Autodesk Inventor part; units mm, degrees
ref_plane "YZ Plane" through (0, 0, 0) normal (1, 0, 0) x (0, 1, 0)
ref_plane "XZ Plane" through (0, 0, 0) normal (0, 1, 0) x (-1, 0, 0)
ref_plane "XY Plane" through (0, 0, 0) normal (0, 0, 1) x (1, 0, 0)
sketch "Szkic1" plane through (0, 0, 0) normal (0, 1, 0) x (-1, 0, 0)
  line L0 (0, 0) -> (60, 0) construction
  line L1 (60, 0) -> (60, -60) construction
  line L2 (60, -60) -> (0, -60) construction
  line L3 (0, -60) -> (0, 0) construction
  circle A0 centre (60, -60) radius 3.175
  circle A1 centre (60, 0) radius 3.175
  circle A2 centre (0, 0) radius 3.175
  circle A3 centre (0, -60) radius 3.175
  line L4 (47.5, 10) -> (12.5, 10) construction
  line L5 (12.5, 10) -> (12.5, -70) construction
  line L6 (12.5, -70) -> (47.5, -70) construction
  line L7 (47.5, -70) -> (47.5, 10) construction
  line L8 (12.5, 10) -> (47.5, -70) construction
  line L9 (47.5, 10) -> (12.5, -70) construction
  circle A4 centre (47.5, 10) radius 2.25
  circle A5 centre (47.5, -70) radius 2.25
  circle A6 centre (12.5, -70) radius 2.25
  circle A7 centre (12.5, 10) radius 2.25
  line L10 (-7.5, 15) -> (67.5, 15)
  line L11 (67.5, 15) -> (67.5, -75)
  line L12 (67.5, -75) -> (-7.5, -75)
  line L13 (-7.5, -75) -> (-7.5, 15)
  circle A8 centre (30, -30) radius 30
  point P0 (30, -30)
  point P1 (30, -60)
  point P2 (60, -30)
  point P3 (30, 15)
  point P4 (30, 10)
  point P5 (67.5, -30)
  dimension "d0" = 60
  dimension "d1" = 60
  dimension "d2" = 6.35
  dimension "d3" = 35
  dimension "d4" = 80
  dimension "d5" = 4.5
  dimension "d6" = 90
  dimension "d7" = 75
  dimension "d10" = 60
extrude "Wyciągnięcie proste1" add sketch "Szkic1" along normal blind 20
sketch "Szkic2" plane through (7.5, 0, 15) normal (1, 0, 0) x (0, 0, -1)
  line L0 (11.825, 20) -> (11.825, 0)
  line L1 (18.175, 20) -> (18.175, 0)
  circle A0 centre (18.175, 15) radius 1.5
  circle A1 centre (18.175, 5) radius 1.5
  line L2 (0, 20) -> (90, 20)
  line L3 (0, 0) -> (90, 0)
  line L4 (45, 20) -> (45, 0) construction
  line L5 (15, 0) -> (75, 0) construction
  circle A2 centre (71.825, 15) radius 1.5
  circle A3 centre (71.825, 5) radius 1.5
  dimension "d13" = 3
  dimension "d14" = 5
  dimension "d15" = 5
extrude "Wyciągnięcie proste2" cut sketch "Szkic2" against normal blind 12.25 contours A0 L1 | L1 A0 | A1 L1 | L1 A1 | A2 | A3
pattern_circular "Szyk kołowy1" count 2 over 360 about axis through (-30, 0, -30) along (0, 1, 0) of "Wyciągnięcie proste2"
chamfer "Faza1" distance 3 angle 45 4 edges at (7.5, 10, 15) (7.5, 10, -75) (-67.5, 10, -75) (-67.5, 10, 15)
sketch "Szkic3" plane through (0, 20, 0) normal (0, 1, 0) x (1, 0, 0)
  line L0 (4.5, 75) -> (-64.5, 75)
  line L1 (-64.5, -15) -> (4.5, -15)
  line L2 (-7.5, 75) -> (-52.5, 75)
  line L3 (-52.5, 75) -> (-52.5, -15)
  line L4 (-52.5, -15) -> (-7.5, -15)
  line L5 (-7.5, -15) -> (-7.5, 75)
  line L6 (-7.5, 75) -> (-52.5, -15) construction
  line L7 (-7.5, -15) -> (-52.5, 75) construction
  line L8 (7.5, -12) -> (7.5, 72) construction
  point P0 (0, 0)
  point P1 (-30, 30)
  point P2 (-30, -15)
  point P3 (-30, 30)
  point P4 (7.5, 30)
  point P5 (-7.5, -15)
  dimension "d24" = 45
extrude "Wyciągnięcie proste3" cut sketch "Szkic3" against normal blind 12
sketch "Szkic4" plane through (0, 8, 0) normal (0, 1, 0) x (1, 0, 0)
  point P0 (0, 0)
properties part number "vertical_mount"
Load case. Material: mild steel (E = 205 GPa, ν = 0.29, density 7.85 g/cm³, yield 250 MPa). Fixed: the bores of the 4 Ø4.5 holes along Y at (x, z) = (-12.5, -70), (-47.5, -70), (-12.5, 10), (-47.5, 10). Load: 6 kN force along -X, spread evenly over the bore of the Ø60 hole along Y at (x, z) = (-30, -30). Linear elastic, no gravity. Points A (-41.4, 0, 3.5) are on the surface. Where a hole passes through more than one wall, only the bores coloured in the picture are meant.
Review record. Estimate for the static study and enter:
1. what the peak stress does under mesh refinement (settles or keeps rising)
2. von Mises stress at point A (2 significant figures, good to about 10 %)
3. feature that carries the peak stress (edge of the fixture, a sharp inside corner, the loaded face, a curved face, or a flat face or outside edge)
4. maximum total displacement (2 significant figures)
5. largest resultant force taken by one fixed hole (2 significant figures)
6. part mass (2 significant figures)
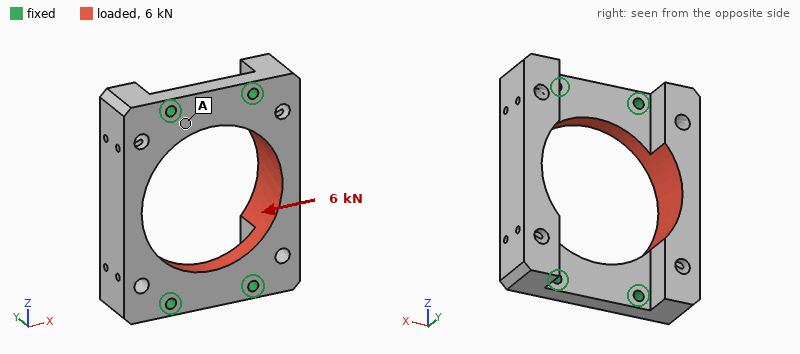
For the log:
keeps rising
11 MPa
edge of the fixture
16 µm
1.6 kN
430 g
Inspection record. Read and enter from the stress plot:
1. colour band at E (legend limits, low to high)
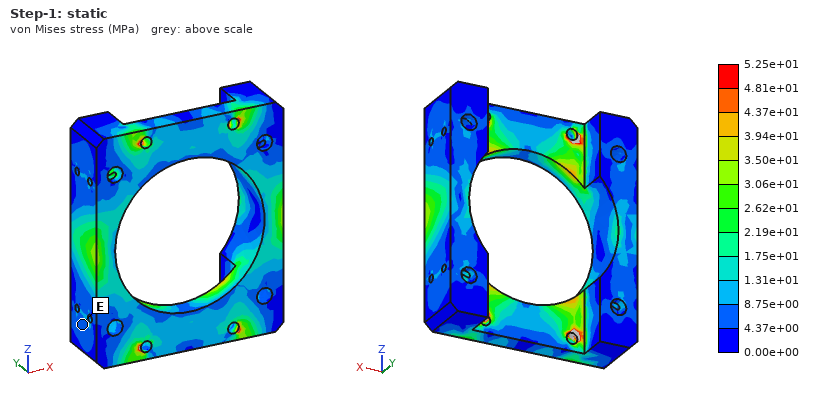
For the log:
4.37e+00 to 8.75e+00 MPa
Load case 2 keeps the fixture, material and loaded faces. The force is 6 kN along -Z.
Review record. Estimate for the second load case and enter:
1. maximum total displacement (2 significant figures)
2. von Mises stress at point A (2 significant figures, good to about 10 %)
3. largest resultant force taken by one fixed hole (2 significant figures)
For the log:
3.0 µm
3.8 MPa
1.5 kN
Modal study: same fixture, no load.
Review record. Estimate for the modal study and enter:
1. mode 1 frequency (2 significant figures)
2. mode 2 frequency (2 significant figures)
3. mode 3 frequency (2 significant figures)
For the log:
4700 Hz
4700 Hz
9400 Hz
